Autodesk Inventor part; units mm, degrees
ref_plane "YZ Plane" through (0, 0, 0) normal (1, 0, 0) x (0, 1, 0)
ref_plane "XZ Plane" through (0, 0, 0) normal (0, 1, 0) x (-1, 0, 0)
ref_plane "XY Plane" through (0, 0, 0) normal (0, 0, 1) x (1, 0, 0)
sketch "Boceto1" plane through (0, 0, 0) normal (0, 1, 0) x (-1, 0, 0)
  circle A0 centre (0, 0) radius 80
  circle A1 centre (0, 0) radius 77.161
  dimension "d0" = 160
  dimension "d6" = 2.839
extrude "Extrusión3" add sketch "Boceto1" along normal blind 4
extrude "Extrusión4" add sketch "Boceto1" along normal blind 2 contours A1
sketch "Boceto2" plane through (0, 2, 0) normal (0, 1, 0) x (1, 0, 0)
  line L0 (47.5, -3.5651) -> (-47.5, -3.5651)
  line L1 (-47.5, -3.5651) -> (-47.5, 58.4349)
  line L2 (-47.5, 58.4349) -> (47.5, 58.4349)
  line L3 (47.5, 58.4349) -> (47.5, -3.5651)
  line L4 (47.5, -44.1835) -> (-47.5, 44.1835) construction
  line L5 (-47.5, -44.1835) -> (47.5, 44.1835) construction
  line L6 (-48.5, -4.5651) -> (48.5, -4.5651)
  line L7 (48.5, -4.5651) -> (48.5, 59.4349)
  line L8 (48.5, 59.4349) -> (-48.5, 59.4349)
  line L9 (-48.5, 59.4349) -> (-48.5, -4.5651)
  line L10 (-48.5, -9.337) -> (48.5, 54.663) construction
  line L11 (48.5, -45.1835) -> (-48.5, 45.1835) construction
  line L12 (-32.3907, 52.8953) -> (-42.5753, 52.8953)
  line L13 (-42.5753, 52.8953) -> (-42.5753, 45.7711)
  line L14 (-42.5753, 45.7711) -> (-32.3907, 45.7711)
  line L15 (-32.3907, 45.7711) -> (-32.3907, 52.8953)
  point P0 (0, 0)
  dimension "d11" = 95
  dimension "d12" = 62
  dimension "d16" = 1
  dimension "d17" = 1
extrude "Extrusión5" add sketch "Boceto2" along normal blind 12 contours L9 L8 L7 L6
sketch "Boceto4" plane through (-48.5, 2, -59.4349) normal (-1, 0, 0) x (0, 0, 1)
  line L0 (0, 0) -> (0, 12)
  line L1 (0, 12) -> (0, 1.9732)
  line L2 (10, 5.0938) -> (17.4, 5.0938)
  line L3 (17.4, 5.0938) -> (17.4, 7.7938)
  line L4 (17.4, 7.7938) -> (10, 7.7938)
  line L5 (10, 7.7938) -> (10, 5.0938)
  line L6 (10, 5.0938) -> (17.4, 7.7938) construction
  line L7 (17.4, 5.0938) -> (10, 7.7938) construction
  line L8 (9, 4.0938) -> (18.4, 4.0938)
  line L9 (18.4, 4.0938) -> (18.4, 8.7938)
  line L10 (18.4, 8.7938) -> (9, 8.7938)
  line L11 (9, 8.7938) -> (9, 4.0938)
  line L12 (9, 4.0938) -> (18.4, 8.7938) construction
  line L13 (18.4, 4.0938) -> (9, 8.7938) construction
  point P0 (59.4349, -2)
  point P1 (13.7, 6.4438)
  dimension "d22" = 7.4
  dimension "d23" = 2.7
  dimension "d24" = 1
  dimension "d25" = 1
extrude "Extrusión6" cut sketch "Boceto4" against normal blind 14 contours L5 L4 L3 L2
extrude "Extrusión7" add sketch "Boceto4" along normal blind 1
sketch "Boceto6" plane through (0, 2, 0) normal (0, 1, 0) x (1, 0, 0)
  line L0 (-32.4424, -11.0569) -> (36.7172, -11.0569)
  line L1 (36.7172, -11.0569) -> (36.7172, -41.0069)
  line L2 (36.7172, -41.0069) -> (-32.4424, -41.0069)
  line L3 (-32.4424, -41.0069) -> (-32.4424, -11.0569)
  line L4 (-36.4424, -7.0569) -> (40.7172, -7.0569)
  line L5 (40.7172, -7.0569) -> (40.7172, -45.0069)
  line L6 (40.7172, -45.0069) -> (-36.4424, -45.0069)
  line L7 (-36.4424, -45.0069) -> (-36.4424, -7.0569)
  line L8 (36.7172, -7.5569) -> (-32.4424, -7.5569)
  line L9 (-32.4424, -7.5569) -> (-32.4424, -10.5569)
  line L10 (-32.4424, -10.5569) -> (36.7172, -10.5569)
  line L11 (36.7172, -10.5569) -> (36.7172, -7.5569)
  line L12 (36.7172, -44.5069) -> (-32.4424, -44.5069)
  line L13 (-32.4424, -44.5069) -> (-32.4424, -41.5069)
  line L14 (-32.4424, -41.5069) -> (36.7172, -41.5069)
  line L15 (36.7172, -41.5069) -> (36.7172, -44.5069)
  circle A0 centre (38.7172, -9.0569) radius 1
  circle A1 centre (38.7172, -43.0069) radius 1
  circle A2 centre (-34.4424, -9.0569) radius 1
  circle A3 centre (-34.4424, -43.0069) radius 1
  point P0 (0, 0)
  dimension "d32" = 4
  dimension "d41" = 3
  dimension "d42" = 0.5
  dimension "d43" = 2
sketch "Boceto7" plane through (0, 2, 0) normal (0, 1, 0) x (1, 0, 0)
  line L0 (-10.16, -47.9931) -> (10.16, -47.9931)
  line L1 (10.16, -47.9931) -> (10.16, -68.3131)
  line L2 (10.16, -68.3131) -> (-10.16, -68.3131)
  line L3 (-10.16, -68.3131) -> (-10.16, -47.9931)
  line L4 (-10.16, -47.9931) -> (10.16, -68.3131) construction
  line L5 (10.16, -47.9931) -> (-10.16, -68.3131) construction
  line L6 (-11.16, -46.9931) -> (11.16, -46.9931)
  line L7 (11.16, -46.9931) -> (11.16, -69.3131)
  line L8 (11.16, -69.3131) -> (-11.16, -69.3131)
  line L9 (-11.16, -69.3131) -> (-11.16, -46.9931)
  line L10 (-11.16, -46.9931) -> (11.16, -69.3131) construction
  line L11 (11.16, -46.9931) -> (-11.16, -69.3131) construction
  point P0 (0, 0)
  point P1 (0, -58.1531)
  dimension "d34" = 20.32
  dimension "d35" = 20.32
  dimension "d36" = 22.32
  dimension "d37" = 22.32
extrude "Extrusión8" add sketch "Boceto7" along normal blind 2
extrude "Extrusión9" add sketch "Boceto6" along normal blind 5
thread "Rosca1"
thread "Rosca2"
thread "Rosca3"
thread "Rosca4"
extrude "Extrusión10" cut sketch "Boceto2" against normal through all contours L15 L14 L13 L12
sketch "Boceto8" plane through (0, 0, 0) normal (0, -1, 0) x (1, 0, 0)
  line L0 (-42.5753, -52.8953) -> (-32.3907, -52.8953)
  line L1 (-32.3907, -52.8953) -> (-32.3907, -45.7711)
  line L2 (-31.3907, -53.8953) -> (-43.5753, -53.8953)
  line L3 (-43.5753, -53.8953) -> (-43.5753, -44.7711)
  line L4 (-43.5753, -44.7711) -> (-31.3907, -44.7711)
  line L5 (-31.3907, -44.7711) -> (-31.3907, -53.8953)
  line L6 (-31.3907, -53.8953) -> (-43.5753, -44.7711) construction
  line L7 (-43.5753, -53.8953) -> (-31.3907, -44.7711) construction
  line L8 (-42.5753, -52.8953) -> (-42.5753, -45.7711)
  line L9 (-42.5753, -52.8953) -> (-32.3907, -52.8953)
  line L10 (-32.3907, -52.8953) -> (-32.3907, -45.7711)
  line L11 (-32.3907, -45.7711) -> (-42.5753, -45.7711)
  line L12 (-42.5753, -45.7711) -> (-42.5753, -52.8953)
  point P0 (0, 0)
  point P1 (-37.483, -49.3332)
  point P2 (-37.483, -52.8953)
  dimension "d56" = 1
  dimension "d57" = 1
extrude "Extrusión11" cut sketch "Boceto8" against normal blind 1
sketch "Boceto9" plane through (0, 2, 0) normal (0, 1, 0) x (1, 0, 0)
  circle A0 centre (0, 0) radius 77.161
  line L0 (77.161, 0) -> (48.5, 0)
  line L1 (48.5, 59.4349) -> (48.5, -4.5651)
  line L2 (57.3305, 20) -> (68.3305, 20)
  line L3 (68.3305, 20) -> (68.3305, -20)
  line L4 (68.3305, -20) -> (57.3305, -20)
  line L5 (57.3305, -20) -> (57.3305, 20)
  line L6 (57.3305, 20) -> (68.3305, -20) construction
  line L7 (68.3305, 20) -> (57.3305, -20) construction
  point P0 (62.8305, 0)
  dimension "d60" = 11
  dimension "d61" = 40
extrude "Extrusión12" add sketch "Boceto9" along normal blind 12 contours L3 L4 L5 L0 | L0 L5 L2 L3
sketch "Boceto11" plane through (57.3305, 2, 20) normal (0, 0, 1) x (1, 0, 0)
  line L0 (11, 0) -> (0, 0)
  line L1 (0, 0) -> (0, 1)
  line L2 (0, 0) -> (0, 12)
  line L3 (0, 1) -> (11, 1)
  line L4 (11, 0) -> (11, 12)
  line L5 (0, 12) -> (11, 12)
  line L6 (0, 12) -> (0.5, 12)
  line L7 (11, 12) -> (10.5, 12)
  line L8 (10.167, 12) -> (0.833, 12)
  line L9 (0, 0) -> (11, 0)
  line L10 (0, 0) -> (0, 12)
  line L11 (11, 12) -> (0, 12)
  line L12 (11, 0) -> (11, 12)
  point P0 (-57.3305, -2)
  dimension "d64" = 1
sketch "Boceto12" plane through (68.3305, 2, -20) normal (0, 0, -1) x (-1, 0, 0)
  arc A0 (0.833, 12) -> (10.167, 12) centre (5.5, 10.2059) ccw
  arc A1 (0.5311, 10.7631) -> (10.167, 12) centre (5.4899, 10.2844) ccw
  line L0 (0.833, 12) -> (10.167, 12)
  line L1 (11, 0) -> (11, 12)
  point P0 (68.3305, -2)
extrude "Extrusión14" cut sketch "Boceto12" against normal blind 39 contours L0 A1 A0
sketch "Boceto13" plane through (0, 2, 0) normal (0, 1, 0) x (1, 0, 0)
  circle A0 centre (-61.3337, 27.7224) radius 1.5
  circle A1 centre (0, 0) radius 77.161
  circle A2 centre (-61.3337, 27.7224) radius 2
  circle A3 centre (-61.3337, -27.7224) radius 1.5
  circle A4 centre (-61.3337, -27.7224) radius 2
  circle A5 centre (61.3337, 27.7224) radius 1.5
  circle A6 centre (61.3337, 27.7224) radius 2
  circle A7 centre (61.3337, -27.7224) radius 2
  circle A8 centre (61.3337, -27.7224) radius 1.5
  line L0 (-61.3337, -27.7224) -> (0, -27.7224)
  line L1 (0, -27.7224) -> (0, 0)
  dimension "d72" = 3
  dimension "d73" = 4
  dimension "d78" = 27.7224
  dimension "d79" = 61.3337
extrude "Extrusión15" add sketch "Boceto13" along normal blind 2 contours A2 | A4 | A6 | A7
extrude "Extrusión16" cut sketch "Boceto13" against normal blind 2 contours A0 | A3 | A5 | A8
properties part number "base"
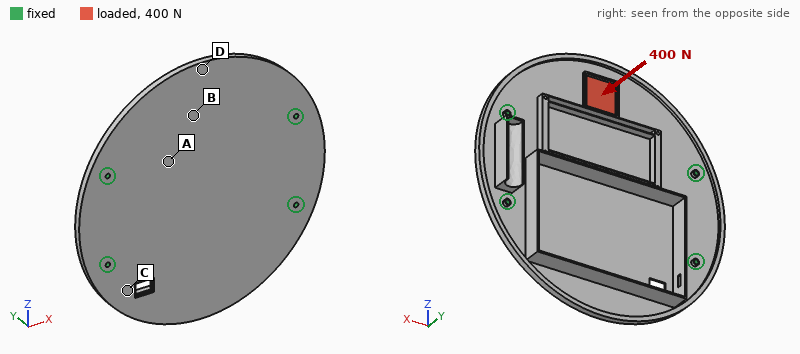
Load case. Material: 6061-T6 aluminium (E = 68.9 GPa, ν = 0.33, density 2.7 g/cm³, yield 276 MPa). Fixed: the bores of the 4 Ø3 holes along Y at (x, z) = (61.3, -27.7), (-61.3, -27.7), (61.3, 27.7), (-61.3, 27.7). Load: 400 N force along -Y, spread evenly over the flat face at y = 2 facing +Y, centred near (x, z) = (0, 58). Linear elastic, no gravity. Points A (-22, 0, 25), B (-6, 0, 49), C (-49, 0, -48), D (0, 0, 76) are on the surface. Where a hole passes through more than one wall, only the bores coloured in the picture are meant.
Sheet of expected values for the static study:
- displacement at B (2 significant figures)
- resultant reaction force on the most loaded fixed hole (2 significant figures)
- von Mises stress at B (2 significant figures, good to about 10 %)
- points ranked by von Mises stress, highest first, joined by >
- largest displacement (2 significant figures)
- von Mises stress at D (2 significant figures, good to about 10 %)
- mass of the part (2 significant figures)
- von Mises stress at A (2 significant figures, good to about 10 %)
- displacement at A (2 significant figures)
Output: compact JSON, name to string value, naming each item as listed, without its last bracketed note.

{"displacement at B": "1.1 mm", "resultant reaction force on the most loaded fixed hole": "360 N", "von Mises stress at B": "62 MPa", "points ranked by von Mises stress, highest first, joined by >": "D > B > A > C", "largest displacement": "2.1 mm", "von Mises stress at D": "77 MPa", "mass of the part": "140 g", "von Mises stress at A": "30 MPa", "displacement at A": "0.39 mm"}
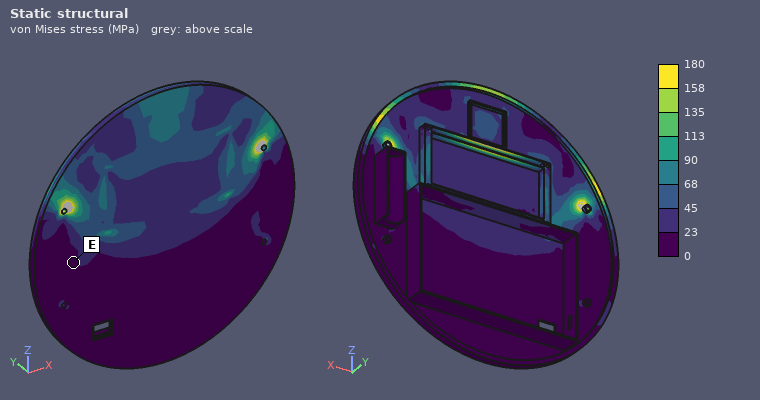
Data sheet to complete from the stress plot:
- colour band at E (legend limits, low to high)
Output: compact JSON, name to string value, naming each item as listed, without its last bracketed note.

{"colour band at E": "0 to 23 MPa"}
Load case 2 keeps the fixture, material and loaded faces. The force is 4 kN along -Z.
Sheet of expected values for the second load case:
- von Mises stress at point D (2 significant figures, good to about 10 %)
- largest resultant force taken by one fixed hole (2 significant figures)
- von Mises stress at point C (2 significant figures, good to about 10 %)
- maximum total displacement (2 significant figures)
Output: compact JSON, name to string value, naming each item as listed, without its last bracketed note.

{"von Mises stress at point D": "66 MPa", "largest resultant force taken by one fixed hole": "1.1 kN", "von Mises stress at point C": "10 MPa", "maximum total displacement": "0.70 mm"}
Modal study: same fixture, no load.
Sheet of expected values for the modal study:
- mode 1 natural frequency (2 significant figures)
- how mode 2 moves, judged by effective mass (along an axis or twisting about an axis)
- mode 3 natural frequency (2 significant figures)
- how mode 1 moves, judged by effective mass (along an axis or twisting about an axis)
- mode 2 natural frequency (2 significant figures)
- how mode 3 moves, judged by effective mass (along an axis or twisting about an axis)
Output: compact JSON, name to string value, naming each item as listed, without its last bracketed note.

{"mode 1 natural frequency": "600 Hz", "how mode 2 moves, judged by effective mass": "along Y", "mode 3 natural frequency": "1200 Hz", "how mode 1 moves, judged by effective mass": "along Y", "mode 2 natural frequency": "900 Hz", "how mode 3 moves, judged by effective mass": "along Y"}
